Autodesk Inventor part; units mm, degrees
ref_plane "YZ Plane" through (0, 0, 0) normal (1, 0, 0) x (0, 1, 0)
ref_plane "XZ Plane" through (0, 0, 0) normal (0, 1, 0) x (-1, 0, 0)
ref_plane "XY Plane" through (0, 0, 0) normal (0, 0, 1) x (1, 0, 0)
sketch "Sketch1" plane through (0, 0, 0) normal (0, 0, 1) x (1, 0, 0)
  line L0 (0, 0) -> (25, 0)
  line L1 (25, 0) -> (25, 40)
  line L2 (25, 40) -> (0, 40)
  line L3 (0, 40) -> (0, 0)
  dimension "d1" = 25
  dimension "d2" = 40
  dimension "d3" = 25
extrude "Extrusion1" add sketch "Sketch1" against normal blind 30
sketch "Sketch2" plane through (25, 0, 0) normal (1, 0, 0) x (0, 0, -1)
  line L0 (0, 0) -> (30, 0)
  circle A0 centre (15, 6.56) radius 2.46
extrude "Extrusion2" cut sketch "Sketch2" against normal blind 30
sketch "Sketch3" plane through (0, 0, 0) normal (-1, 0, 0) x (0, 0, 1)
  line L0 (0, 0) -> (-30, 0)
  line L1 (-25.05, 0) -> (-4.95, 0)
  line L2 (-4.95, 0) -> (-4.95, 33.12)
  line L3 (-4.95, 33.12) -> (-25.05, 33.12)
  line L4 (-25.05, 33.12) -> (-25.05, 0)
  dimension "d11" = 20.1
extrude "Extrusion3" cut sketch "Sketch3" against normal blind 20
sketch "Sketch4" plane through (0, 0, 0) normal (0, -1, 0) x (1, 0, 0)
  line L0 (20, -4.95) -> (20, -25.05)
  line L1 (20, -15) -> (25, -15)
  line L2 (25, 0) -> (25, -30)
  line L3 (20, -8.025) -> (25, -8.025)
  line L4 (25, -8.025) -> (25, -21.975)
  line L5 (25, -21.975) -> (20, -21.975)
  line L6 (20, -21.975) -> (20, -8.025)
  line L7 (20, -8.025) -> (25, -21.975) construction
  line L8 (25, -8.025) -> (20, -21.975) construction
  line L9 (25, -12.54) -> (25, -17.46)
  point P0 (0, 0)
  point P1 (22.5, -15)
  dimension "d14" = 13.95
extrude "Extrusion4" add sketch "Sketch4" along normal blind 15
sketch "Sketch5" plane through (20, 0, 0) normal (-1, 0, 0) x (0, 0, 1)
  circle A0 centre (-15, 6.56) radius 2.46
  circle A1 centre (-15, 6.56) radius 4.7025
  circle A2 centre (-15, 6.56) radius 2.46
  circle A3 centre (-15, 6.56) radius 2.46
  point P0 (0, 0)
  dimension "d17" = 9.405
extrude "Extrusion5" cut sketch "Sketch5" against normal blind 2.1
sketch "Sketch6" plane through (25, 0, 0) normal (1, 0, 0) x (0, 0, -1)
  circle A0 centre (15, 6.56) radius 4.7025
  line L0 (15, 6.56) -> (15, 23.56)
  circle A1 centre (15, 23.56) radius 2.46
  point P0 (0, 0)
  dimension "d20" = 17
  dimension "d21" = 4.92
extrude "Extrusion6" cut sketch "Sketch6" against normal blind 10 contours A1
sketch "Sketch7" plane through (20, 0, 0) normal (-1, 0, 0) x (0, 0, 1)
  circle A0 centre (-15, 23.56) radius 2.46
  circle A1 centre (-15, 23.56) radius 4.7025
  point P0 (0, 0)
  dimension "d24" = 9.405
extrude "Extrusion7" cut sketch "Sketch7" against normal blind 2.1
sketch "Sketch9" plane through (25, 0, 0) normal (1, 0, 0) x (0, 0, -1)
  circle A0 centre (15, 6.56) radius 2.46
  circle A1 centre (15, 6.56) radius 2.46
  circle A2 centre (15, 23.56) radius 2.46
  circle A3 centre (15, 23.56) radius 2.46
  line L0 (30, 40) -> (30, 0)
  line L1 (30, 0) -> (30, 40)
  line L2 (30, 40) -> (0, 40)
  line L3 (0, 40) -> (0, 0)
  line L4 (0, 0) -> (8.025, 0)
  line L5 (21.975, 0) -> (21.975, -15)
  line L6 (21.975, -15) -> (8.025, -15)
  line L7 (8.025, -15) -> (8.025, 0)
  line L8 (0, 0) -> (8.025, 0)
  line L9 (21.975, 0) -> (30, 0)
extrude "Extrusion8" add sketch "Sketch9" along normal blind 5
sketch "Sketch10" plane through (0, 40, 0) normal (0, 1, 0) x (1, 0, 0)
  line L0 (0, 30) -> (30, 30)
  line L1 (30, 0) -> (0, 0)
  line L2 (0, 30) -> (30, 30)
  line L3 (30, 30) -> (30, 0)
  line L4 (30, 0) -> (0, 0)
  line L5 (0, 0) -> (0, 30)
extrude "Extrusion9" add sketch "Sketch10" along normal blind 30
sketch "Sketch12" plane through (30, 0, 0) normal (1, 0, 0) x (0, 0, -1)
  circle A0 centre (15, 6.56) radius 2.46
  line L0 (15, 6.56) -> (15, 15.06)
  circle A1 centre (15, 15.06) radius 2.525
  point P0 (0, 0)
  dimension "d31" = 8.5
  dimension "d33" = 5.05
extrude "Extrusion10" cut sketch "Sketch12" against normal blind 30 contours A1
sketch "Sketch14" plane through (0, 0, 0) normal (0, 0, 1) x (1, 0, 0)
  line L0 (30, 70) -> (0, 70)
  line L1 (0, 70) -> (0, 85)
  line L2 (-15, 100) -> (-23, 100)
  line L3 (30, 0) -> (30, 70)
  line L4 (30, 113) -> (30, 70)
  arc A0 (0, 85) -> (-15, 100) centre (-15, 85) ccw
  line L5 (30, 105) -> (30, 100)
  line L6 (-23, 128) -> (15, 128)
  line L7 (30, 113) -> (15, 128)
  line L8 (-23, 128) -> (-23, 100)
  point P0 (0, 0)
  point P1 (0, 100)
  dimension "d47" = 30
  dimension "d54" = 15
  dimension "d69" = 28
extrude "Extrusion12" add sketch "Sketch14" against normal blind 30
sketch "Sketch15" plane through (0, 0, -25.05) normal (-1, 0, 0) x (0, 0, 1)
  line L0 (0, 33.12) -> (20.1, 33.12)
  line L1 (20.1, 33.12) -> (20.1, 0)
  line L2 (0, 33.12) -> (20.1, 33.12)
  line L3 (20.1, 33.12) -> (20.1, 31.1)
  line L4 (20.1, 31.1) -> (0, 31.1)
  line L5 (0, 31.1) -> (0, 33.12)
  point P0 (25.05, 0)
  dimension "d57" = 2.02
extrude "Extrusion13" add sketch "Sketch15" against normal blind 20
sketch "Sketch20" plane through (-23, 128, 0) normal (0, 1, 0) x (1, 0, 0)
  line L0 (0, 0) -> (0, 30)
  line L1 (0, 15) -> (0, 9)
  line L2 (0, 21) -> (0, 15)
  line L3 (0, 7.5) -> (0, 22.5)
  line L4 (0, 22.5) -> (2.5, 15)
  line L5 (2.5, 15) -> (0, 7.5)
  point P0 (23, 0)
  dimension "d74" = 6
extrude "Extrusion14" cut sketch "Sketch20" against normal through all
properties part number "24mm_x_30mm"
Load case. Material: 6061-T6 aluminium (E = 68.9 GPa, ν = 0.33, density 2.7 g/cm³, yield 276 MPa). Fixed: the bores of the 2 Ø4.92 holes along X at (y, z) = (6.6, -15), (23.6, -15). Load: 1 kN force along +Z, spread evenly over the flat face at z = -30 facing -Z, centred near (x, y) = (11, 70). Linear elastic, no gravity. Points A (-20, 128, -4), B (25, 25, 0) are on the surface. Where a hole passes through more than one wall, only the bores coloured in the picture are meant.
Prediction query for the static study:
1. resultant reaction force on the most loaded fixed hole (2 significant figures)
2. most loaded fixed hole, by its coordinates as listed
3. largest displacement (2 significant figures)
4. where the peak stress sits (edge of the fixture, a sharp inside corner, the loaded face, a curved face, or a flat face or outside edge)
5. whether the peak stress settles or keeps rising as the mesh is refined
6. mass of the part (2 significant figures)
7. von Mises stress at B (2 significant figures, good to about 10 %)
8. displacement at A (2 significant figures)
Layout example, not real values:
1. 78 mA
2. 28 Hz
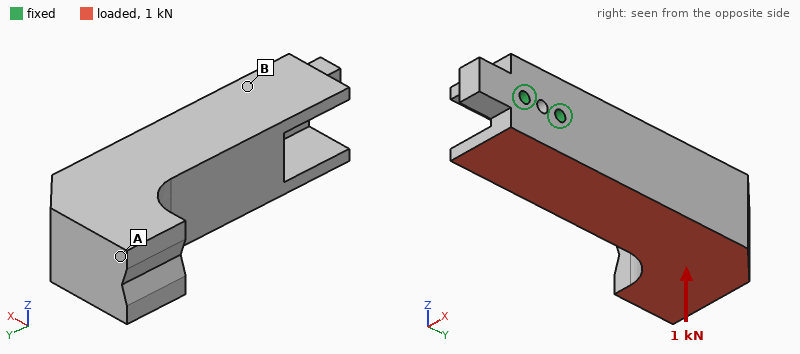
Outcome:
1. 3.0 kN
2. (23.6, -15)
3. 0.12 mm
4. edge of the fixture
5. keeps rising
6. 330 g
7. 21 MPa
8. 0.12 mm
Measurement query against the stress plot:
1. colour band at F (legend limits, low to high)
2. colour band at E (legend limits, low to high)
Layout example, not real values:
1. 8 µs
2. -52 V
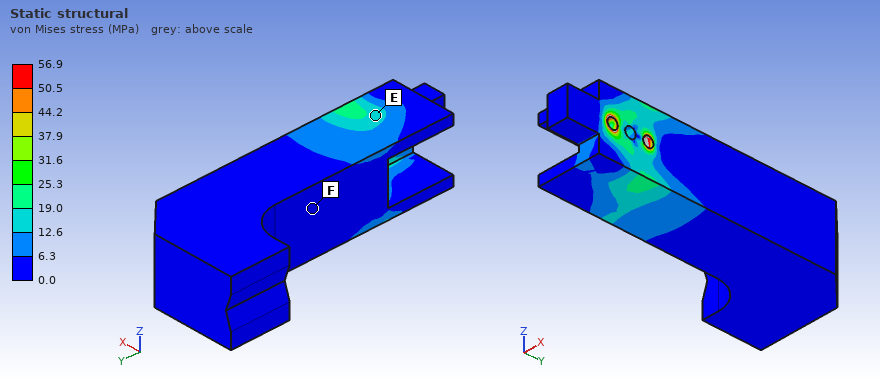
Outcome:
1. 0.0 to 6.3 MPa
2. 12.6 to 19.0 MPa
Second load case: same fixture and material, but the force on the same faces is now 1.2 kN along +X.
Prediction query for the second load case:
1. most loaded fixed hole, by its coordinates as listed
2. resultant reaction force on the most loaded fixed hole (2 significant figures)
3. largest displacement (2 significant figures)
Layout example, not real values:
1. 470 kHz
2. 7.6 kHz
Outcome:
1. (23.6, -15)
2. 3.3 kN
3. 0.20 mm
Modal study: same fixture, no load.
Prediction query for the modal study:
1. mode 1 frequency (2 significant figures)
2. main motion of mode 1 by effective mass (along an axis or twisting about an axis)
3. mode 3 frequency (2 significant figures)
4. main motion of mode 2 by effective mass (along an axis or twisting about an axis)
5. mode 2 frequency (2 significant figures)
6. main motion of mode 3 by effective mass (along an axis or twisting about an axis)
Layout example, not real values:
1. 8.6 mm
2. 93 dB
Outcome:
1. 820 Hz
2. along X
3. 2600 Hz
4. along Z
5. 960 Hz
6. twisting about Y
